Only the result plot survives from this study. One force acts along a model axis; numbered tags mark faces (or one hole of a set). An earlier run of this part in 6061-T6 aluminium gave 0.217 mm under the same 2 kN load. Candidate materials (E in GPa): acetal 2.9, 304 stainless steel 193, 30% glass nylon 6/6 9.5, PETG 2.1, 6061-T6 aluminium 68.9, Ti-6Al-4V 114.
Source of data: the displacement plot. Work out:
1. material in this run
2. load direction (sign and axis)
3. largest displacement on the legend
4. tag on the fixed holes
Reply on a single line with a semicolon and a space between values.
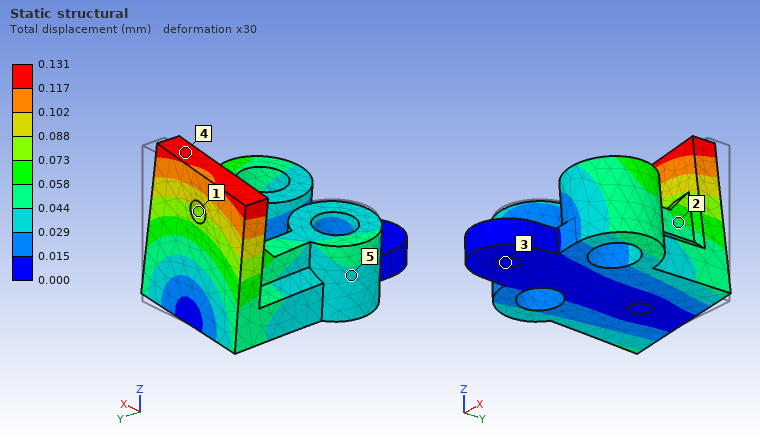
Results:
Ti-6Al-4V; -X; 0.131 mm; 3
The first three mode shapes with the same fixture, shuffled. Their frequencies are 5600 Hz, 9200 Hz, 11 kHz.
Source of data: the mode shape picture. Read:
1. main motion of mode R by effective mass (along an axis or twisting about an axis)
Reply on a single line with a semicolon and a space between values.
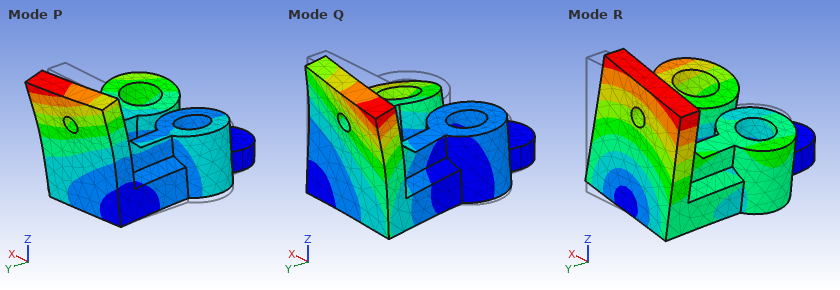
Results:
along X
